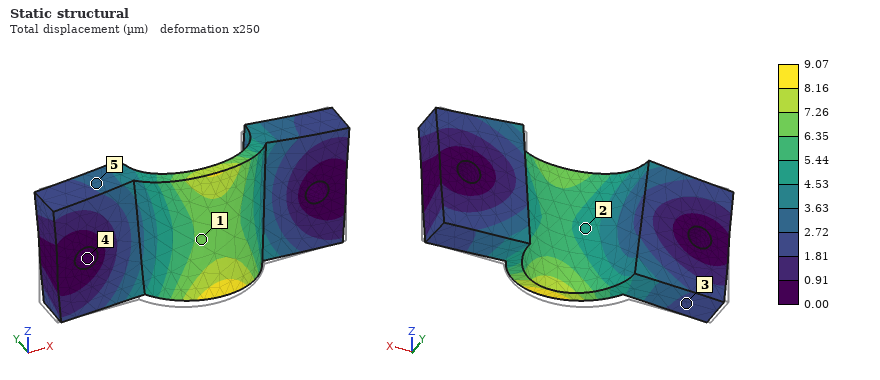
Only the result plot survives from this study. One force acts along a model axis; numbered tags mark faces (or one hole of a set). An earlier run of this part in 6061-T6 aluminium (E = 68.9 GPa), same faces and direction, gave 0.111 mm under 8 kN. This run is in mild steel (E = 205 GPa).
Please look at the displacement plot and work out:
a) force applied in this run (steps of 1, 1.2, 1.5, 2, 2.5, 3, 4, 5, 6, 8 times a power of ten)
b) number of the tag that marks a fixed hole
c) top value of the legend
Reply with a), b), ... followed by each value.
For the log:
a) 2 kN
b) 4
c) 9.07 µm
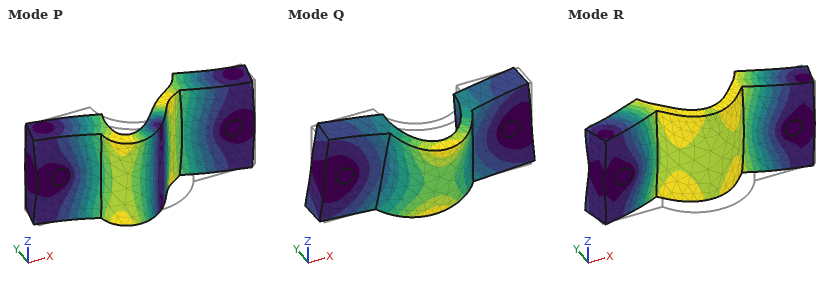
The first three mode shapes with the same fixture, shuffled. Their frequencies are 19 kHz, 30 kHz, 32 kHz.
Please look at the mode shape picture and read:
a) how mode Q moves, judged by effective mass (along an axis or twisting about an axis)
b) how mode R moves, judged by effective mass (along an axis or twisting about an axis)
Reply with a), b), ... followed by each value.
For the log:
a) along Z
b) along Y
